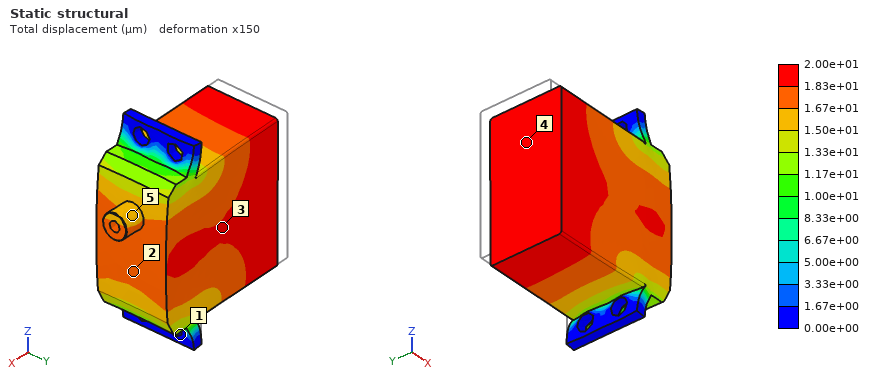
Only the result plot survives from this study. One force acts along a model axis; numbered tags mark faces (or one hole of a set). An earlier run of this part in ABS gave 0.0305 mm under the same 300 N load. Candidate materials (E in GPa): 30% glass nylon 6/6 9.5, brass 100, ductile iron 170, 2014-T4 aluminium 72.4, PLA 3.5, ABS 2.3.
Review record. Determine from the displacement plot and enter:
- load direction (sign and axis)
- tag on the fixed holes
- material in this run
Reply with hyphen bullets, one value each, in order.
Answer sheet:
- +X
- 1
- PLA
